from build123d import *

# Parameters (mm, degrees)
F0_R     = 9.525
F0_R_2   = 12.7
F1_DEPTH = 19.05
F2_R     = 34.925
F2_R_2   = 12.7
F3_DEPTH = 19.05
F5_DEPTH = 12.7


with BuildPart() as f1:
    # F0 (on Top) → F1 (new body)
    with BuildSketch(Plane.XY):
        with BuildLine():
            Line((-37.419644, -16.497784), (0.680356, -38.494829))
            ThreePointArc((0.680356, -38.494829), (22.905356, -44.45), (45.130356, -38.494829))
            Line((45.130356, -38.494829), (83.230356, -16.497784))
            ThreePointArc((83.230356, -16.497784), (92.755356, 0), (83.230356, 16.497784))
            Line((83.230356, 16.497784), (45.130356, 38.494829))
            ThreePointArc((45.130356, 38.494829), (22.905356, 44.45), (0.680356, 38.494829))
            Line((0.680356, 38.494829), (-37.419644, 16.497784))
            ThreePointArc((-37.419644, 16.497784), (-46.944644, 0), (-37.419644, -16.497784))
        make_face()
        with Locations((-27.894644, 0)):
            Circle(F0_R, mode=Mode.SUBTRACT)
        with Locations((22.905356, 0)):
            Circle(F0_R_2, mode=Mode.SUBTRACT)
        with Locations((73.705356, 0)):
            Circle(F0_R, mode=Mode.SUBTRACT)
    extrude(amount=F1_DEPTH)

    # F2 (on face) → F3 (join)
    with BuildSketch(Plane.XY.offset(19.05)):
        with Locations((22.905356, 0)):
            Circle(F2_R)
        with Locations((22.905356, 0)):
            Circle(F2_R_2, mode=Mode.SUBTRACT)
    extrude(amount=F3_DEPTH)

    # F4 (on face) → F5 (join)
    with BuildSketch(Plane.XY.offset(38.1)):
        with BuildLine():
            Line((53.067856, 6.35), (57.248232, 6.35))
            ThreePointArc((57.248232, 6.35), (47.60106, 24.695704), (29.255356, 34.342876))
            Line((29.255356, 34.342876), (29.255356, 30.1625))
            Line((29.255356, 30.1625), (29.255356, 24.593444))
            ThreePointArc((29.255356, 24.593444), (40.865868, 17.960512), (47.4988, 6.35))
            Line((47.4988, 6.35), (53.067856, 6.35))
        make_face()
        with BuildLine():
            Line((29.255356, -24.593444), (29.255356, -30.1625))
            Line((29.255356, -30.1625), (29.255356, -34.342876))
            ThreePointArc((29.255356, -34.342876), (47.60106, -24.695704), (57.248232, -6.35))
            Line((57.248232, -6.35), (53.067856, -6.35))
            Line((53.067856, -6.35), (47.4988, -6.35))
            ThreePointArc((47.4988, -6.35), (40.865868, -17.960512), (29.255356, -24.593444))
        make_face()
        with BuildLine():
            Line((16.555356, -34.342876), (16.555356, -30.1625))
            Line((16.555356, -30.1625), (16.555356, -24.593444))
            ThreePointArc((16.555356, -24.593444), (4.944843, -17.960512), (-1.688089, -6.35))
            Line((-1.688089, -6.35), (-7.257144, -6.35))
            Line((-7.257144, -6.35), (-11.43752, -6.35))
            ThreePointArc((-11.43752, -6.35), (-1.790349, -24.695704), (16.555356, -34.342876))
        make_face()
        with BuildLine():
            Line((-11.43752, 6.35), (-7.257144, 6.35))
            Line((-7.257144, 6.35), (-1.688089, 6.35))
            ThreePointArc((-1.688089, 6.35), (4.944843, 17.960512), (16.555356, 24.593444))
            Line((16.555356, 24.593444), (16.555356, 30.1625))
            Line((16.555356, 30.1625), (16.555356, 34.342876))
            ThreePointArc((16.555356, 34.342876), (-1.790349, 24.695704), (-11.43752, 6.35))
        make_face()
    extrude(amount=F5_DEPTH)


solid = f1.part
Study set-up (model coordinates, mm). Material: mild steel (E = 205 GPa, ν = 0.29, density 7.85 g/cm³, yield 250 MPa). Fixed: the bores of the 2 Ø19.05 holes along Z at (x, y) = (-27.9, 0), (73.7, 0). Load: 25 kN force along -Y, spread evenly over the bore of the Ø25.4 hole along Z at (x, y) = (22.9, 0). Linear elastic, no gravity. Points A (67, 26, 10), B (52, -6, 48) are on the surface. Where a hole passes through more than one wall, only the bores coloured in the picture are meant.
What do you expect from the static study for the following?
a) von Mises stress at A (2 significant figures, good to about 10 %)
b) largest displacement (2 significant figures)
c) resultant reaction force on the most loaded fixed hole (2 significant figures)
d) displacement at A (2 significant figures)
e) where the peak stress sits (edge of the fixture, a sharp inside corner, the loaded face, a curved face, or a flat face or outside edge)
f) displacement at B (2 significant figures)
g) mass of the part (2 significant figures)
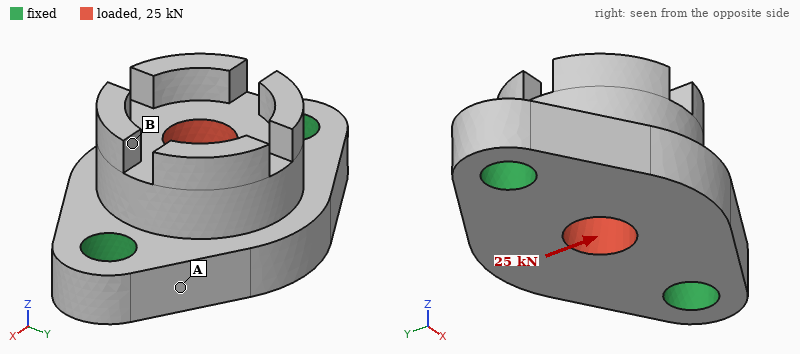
19 MPa
18 µm
13 kN
3.3 µm
edge of the fixture
14 µm
1.7 kg
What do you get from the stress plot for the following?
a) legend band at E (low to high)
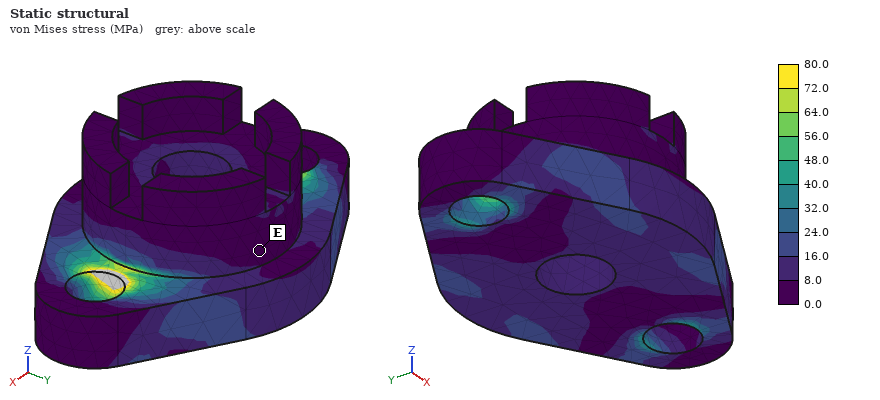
0.0 to 8.0 MPa
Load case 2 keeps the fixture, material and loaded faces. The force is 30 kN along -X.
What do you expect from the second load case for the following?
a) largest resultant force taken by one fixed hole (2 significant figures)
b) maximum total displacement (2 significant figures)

15 kN
4.5 µm
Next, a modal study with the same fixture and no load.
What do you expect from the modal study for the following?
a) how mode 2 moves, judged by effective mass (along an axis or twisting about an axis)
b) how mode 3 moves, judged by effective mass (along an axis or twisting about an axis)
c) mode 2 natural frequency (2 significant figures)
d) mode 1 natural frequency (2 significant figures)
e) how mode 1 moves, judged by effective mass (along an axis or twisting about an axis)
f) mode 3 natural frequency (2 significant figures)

along Z
along Y
7300 Hz
4700 Hz
along Y
11 kHz
